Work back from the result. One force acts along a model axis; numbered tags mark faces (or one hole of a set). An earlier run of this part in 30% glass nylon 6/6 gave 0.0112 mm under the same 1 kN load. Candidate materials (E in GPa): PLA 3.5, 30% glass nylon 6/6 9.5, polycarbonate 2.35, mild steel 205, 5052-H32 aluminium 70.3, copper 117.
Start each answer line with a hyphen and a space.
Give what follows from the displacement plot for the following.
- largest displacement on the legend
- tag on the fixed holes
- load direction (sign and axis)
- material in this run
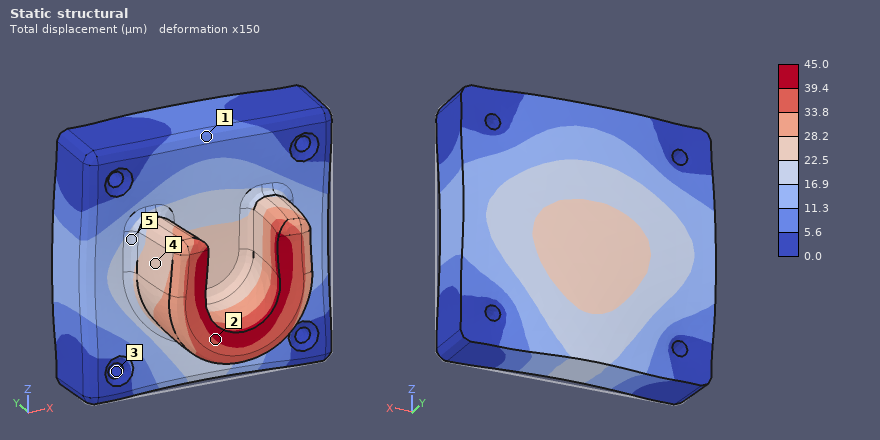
- 45.0 µm
- 3
- +Y
- polycarbonate
